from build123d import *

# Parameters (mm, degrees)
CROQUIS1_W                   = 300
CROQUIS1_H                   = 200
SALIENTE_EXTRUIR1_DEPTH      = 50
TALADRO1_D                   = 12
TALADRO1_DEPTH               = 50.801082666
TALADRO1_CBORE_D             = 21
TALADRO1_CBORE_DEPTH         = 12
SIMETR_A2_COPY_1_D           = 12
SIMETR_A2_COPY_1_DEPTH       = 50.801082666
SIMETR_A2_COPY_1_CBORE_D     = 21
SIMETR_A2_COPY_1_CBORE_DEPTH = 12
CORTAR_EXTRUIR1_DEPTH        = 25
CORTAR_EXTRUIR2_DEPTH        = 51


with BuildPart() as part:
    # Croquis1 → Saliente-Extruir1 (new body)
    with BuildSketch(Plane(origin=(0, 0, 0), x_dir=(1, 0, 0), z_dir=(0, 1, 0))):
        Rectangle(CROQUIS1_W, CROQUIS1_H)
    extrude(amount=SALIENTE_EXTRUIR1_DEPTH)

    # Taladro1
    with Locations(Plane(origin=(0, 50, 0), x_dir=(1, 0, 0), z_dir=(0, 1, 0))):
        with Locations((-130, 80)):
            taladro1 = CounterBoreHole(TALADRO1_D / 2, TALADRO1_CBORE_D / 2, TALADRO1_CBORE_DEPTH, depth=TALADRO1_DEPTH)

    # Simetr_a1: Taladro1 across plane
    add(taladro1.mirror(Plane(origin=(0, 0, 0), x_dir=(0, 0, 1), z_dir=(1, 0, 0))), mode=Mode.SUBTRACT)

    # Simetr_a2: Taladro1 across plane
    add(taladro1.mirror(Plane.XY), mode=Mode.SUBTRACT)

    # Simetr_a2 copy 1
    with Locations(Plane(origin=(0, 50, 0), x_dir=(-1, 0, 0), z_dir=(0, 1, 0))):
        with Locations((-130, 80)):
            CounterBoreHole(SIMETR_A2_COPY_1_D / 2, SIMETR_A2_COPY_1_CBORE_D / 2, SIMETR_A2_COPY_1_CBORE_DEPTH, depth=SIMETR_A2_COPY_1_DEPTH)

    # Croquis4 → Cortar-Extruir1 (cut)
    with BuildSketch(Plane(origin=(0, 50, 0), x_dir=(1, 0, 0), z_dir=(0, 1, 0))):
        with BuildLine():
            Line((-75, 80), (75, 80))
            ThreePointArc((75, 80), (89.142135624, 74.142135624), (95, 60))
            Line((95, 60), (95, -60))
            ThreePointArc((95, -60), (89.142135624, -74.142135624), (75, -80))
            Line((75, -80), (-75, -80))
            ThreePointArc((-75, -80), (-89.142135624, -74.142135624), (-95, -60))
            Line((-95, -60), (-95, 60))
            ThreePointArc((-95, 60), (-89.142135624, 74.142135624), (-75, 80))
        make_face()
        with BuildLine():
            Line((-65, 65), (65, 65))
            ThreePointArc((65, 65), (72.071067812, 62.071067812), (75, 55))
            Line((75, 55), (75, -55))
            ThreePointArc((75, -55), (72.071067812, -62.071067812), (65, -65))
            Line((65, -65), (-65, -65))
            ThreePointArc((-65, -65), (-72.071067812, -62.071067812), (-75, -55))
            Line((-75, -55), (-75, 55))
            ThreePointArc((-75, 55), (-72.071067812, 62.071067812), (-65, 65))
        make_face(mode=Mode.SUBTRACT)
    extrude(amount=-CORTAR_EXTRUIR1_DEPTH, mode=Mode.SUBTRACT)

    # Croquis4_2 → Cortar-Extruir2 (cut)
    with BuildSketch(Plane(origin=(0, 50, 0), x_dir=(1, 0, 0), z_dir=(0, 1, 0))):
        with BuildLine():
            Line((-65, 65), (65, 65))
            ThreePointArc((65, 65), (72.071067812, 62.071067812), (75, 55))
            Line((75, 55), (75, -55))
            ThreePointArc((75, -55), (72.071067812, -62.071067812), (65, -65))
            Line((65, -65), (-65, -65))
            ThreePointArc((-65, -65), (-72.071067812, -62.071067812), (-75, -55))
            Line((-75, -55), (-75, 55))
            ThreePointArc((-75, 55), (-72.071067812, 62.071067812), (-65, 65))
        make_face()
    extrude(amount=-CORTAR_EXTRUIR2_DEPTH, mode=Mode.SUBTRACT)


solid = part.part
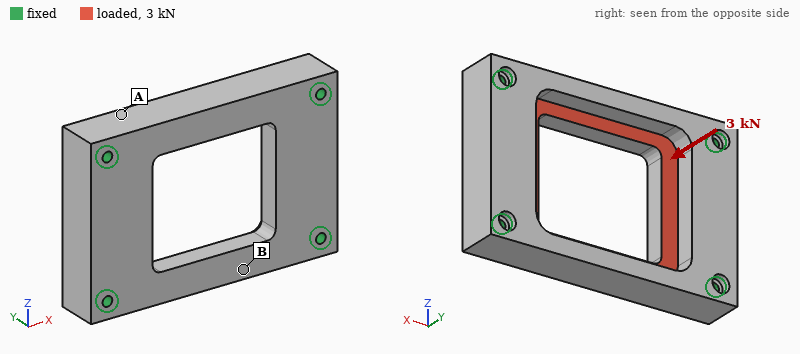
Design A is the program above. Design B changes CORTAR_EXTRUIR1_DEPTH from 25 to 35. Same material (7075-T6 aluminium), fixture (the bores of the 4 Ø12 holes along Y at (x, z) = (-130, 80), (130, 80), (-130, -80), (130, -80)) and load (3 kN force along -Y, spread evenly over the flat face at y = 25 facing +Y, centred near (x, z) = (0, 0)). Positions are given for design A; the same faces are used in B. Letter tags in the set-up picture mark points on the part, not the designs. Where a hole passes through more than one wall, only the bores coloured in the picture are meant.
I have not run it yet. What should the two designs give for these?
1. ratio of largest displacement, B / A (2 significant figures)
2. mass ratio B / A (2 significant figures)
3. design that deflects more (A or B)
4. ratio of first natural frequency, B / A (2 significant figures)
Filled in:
1.2
0.94
B
1.0
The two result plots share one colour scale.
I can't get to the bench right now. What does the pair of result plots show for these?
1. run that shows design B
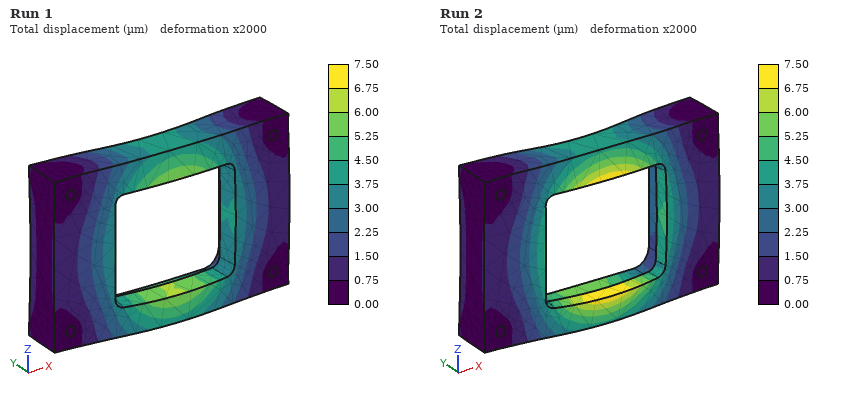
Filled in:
Run 2
